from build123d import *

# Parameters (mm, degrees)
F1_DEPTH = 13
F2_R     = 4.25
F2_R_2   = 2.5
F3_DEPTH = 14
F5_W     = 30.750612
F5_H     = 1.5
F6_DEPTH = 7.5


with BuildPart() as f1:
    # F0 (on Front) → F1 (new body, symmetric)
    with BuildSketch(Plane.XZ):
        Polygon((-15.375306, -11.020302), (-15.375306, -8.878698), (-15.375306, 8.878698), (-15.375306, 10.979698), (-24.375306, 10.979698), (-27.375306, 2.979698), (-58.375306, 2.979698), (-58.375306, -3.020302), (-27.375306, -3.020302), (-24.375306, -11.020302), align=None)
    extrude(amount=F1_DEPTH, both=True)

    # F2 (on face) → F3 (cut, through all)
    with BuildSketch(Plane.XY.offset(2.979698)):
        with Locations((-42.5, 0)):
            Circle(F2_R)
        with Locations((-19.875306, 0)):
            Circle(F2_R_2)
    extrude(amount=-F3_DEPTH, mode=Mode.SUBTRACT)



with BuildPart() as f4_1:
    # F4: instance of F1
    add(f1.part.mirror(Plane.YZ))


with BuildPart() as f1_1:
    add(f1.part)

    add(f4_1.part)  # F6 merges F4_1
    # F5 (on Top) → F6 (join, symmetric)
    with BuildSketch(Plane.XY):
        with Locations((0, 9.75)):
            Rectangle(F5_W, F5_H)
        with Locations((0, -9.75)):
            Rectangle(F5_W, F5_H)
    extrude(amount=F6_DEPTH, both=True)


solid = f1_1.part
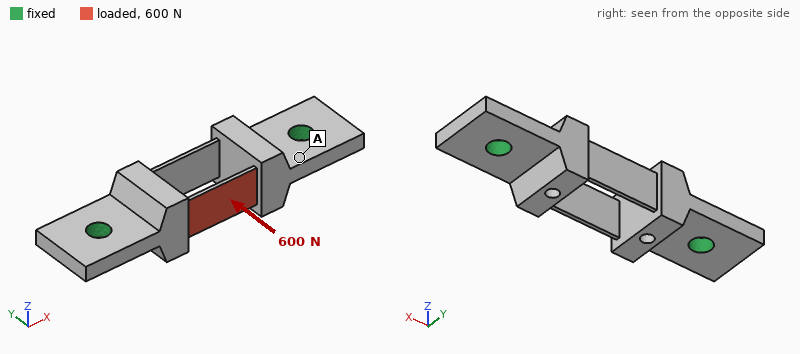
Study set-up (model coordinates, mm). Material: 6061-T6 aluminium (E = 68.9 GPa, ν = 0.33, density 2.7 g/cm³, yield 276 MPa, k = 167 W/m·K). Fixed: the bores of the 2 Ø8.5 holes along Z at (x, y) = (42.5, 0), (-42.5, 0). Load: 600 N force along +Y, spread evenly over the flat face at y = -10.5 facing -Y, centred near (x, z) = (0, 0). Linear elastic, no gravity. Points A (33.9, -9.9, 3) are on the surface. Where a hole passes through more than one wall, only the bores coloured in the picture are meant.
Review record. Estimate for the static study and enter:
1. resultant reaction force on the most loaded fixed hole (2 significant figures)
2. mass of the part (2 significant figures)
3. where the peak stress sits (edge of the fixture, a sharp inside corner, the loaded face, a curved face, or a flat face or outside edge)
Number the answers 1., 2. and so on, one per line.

1. 300 N
2. 60 g
3. a flat face or outside edge
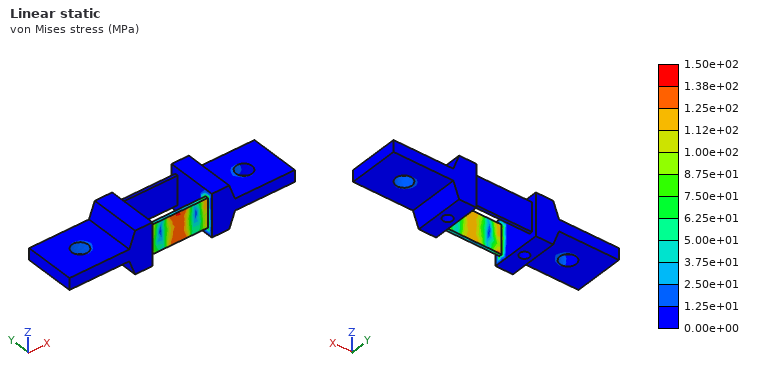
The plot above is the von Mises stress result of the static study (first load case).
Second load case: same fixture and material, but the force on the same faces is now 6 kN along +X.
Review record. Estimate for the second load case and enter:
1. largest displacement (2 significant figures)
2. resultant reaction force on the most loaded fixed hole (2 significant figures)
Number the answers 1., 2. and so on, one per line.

1. 42 µm
2. 3.0 kN
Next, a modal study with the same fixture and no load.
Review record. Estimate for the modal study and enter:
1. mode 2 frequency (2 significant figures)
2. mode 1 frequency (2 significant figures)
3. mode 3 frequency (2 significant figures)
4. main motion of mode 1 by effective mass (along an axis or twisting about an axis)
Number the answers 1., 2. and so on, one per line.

1. 7300 Hz
2. 5200 Hz
3. 7600 Hz
4. along Z
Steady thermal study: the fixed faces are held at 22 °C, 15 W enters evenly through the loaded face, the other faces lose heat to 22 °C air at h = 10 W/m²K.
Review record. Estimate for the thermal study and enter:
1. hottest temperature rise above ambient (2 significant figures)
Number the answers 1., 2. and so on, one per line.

1. 24 K
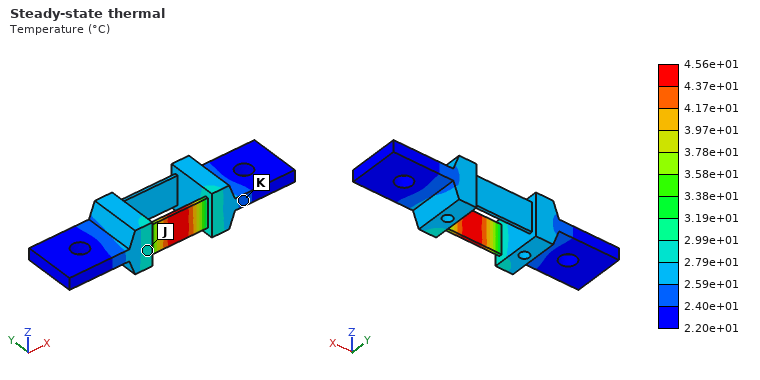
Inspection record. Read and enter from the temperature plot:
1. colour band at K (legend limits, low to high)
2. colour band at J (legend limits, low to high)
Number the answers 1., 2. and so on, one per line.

1. 2.40e+01 to 2.59e+01 °C
2. 2.79e+01 to 2.99e+01 °C
